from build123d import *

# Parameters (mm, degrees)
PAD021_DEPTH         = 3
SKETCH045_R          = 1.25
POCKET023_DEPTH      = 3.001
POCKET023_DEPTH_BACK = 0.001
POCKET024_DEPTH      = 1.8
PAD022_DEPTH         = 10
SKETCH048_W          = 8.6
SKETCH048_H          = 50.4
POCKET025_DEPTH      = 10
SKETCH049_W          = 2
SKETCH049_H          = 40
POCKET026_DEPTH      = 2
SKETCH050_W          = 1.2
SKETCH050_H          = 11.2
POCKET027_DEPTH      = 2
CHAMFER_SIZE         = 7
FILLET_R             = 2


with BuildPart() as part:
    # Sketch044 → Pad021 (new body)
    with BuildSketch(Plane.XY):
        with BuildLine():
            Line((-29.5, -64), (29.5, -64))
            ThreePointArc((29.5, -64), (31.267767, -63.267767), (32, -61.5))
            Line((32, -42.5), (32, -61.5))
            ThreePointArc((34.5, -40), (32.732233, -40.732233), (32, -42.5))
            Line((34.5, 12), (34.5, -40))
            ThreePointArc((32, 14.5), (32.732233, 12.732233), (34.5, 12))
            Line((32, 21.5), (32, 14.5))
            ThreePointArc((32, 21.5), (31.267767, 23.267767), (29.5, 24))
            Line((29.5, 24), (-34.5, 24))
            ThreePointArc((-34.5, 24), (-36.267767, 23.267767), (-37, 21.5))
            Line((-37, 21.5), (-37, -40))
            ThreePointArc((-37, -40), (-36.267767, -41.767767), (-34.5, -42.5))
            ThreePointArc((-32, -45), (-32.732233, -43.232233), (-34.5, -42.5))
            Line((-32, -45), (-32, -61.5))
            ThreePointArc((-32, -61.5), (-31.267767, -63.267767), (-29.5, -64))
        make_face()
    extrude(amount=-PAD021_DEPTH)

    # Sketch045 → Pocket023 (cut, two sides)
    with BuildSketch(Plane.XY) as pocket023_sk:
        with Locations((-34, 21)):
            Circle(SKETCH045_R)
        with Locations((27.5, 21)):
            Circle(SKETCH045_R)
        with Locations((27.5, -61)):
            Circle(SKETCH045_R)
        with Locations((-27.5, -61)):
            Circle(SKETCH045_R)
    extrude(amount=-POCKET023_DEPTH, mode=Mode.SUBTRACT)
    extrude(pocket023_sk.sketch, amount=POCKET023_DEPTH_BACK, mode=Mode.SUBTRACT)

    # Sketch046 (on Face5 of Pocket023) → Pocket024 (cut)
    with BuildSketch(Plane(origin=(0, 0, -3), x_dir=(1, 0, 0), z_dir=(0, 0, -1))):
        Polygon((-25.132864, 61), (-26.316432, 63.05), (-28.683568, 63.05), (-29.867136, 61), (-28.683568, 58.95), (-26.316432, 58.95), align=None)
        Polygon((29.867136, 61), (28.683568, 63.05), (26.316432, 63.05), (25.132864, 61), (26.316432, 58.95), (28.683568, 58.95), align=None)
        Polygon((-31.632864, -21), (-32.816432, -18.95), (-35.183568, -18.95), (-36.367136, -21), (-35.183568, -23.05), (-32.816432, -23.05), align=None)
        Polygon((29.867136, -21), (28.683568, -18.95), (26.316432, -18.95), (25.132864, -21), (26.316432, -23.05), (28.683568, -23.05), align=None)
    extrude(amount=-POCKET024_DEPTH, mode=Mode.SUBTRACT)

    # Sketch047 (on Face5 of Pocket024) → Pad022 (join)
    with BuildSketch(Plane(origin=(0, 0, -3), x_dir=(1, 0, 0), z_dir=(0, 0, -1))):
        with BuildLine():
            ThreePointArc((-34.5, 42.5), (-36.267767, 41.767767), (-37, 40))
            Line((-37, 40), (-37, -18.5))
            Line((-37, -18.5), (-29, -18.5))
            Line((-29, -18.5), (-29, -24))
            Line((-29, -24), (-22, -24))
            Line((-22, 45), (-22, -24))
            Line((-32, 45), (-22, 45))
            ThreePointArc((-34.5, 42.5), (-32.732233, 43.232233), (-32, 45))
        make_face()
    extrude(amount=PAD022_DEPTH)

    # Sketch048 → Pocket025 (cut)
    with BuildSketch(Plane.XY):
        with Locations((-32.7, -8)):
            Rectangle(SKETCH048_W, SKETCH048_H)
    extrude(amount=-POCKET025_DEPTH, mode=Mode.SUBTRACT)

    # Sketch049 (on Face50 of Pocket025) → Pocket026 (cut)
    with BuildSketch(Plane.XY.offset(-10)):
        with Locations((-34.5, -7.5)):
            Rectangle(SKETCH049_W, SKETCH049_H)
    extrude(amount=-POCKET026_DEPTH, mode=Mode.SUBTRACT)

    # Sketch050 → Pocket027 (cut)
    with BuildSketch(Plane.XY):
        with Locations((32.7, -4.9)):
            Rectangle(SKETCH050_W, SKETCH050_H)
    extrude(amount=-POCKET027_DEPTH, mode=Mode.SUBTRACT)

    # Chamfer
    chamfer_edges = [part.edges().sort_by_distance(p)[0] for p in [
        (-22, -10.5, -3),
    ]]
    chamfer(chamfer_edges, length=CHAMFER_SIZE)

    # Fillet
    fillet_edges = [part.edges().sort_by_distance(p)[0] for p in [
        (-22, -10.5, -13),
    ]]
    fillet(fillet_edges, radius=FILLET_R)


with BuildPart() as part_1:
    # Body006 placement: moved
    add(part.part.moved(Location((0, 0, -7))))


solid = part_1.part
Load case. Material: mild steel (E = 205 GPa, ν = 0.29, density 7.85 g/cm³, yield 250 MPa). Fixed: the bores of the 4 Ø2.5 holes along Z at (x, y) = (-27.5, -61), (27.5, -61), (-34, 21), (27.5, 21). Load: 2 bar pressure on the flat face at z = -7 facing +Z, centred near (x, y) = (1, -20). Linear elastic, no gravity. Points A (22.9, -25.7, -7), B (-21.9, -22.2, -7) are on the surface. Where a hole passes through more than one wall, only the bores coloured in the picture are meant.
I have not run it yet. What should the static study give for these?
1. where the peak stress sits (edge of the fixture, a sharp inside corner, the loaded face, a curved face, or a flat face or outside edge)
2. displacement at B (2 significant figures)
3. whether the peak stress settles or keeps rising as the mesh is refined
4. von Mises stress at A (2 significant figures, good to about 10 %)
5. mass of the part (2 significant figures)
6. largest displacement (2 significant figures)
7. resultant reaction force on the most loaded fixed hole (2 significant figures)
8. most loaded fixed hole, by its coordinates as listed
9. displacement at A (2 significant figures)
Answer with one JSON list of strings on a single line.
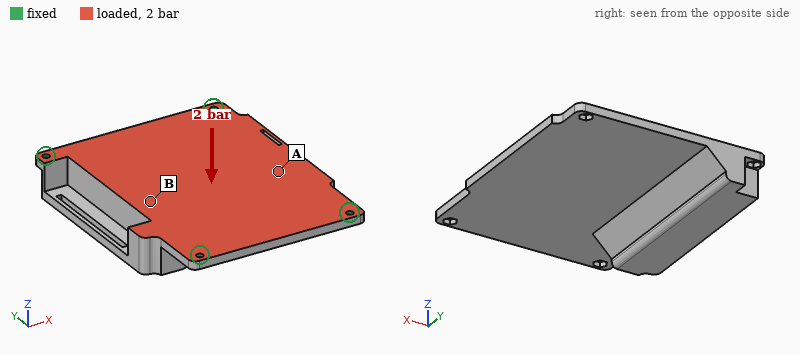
["edge of the fixture", "35 µm", "keeps rising", "37 MPa", "200 g", "95 µm", "770 N", "(27.5, 21)", "90 µm"]
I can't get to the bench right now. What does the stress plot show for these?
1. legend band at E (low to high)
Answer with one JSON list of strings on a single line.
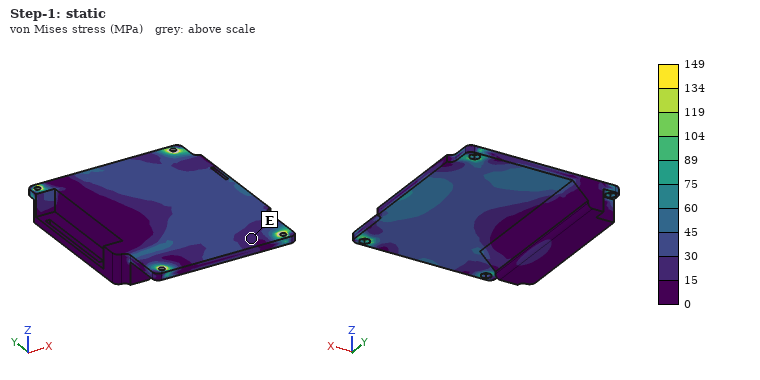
["15 to 30 MPa"]
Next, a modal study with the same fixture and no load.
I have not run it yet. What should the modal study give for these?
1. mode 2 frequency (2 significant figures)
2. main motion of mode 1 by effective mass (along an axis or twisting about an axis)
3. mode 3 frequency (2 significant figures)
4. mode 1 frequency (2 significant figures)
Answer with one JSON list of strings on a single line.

["2800 Hz", "along Z", "3300 Hz", "1700 Hz"]
